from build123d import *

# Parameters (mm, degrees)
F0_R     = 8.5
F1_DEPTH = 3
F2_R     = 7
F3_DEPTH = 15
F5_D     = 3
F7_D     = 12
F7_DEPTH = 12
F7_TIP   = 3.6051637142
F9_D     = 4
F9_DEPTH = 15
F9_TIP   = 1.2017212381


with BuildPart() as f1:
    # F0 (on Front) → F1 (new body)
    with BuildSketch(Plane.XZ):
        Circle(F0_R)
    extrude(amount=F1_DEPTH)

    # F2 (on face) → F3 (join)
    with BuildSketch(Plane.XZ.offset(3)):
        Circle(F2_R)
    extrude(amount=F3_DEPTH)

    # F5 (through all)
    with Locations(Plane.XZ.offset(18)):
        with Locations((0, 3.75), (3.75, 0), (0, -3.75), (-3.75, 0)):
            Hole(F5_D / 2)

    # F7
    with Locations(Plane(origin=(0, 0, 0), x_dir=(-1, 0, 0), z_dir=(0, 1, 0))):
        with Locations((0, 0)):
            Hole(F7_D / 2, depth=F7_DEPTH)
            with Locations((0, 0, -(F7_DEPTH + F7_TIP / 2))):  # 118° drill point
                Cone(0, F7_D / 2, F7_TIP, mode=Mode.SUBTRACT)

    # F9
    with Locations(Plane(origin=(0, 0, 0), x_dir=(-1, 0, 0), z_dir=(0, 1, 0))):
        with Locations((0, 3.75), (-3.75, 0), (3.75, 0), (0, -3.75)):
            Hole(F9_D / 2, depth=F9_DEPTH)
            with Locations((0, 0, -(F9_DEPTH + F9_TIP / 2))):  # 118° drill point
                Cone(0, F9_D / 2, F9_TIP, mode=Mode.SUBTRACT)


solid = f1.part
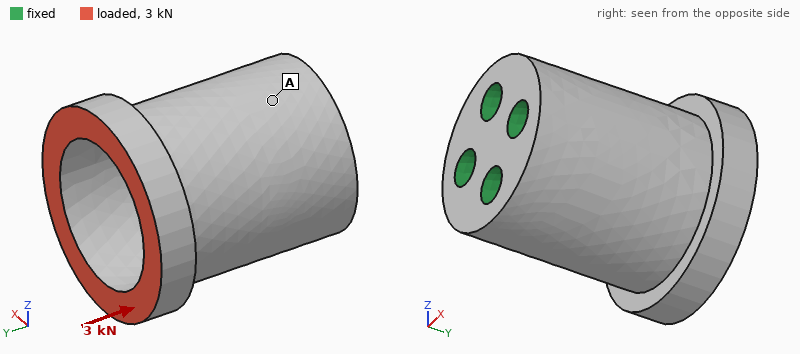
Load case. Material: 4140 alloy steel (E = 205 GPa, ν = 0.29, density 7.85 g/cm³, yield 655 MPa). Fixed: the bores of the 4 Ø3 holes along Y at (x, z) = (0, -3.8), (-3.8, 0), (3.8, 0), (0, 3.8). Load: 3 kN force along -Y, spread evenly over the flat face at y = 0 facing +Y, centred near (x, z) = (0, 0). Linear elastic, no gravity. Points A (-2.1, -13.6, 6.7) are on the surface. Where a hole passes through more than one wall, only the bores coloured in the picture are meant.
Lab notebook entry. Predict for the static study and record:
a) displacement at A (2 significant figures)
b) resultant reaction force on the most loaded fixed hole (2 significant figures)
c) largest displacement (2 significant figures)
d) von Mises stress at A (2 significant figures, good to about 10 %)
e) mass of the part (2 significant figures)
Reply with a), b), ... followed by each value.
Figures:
a) 1.7 µm
b) 750 N
c) 7.3 µm
d) 59 MPa
e) 10 g
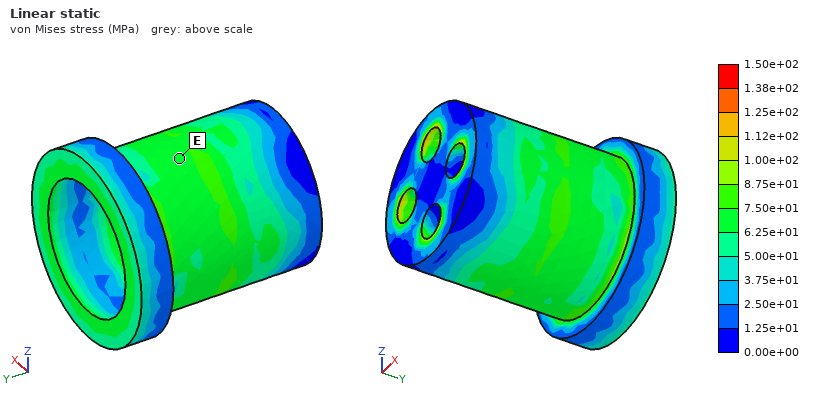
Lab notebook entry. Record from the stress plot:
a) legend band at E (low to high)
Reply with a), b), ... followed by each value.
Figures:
a) 6.25e+01 to 7.50e+01 MPa
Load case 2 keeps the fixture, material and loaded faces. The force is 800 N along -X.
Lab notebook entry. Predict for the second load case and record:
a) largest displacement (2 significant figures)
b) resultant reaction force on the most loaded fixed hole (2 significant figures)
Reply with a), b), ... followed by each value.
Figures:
a) 19 µm
b) 1.0 kN
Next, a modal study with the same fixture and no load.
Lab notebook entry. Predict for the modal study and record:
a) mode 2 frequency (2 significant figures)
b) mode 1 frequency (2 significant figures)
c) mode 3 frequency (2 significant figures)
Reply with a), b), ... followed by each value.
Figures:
a) 20 kHz
b) 20 kHz
c) 28 kHz
